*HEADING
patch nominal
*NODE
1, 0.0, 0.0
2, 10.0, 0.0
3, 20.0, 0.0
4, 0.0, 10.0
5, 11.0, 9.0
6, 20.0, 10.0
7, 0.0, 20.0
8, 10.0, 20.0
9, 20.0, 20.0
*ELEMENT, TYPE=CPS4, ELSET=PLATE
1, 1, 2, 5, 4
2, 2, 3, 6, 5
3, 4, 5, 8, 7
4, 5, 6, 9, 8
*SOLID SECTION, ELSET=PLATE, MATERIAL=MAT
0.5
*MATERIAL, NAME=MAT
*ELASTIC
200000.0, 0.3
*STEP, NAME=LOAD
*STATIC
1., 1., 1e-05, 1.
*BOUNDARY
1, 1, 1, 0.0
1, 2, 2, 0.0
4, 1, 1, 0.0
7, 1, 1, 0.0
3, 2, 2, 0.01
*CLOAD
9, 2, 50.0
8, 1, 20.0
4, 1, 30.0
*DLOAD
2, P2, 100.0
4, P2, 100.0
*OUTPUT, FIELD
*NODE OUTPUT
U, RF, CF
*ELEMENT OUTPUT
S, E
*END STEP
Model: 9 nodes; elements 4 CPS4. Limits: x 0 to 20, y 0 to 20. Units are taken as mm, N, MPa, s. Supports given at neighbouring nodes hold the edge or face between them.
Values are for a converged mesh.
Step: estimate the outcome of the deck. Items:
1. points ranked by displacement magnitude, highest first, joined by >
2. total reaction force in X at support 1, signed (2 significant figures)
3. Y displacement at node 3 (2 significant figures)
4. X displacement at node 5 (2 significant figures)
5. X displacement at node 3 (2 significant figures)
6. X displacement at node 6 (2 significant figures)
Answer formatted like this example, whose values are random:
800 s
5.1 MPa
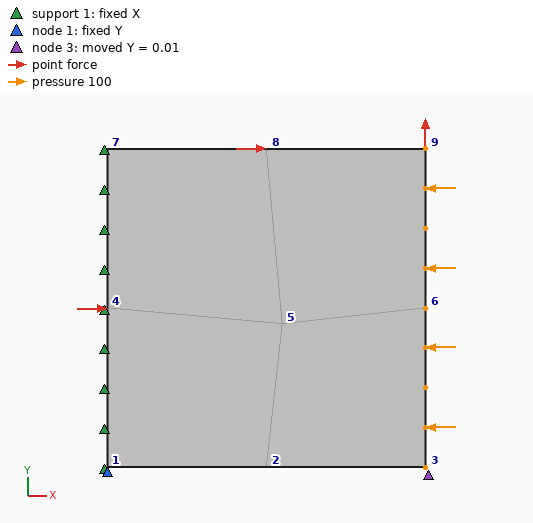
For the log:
node 6 > node 3 > node 8 > node 5 > node 2
950 N
0.010 mm
-0.0055 mm
-0.0066 mm
-0.010 mm
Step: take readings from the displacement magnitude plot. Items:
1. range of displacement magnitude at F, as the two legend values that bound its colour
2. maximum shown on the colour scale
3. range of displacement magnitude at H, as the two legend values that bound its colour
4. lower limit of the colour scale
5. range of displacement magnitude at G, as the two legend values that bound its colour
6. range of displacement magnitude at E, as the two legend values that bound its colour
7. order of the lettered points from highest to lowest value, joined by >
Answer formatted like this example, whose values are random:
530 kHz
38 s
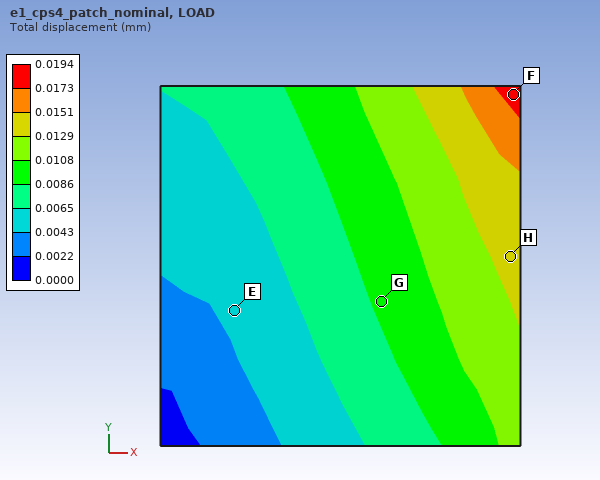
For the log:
0.0173 to 0.0194 mm
0.0194 mm
0.0129 to 0.0151 mm
0.0000 mm
0.0086 to 0.0108 mm
0.0043 to 0.0065 mm
F > H > G > E
